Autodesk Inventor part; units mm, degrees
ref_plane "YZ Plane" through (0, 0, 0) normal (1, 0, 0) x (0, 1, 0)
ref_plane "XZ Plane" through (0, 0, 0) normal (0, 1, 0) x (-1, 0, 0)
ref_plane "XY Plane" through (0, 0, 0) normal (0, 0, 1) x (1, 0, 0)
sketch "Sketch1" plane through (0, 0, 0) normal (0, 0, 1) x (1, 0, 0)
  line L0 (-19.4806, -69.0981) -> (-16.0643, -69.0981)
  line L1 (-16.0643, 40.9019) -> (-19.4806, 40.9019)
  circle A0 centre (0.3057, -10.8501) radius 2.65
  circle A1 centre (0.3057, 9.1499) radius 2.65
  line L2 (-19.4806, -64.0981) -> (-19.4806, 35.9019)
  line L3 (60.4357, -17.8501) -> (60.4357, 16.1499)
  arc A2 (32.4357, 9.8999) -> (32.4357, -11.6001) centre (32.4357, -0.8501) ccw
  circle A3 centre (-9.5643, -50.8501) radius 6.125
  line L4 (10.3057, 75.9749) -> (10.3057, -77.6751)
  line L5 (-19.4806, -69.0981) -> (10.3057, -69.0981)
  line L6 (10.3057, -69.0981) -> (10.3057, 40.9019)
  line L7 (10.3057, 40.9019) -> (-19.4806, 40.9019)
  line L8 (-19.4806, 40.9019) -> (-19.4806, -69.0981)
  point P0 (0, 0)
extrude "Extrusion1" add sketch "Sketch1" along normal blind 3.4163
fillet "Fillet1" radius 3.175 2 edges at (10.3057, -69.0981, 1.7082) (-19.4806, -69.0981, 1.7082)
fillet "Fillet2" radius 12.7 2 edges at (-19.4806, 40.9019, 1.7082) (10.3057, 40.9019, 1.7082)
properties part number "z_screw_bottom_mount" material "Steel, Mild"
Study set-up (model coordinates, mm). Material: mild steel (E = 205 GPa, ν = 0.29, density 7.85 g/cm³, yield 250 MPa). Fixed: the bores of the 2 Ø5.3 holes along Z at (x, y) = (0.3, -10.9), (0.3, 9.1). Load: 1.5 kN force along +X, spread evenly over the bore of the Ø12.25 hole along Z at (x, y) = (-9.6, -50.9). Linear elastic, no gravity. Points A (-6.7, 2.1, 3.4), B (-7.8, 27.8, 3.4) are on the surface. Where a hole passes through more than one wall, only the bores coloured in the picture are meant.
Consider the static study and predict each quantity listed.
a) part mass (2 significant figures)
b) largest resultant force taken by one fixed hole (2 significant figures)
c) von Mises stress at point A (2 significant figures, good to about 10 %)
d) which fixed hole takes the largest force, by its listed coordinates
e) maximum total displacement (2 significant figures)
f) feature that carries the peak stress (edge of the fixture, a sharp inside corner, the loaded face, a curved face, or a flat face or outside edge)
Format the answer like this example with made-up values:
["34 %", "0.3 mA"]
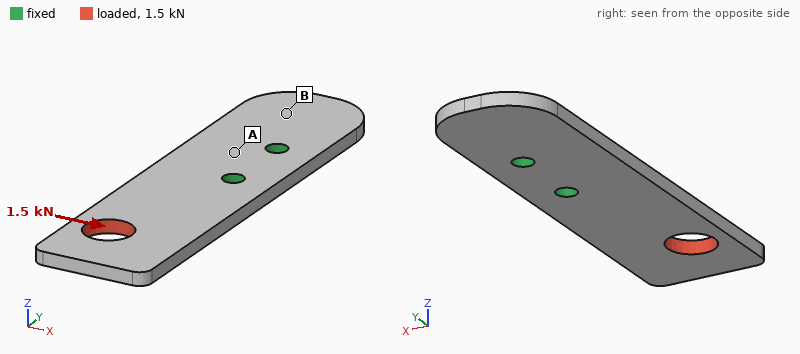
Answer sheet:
["82 g", "3.7 kN", "58 MPa", "(0.3, -10.9)", "82 µm", "edge of the fixture"]
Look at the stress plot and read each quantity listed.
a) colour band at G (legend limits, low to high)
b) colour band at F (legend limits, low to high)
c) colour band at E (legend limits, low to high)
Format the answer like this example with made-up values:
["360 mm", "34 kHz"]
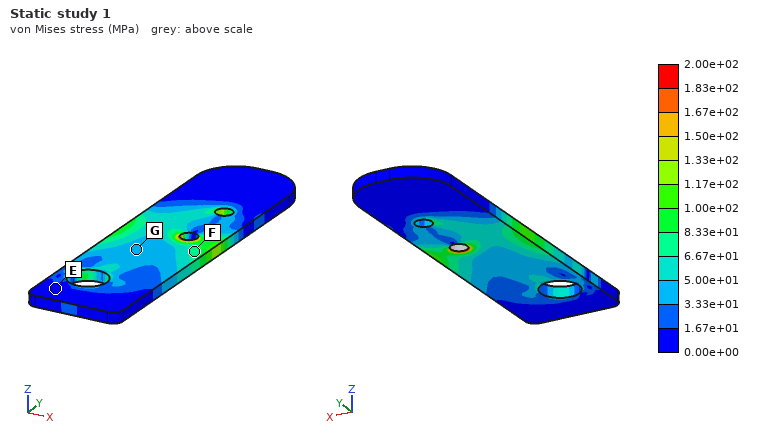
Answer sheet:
["3.33e+01 to 5.00e+01 MPa", "6.67e+01 to 8.33e+01 MPa", "0.00e+00 to 1.67e+01 MPa"]
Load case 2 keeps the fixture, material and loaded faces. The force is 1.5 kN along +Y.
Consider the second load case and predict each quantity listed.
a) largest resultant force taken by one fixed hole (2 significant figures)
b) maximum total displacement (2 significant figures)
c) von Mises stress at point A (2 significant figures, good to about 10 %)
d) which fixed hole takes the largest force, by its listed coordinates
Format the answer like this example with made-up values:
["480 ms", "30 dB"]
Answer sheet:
["1.2 kN", "19 µm", "18 MPa", "(0.3, -10.9)"]
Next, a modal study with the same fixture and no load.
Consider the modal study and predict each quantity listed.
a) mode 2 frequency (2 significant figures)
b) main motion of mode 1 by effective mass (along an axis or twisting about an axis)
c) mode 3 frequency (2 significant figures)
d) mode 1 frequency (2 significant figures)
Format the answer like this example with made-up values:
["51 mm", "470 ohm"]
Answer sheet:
["3000 Hz", "along Z", "3100 Hz", "870 Hz"]
